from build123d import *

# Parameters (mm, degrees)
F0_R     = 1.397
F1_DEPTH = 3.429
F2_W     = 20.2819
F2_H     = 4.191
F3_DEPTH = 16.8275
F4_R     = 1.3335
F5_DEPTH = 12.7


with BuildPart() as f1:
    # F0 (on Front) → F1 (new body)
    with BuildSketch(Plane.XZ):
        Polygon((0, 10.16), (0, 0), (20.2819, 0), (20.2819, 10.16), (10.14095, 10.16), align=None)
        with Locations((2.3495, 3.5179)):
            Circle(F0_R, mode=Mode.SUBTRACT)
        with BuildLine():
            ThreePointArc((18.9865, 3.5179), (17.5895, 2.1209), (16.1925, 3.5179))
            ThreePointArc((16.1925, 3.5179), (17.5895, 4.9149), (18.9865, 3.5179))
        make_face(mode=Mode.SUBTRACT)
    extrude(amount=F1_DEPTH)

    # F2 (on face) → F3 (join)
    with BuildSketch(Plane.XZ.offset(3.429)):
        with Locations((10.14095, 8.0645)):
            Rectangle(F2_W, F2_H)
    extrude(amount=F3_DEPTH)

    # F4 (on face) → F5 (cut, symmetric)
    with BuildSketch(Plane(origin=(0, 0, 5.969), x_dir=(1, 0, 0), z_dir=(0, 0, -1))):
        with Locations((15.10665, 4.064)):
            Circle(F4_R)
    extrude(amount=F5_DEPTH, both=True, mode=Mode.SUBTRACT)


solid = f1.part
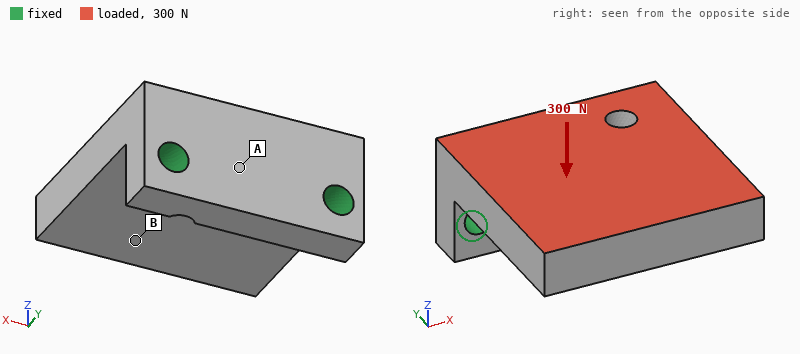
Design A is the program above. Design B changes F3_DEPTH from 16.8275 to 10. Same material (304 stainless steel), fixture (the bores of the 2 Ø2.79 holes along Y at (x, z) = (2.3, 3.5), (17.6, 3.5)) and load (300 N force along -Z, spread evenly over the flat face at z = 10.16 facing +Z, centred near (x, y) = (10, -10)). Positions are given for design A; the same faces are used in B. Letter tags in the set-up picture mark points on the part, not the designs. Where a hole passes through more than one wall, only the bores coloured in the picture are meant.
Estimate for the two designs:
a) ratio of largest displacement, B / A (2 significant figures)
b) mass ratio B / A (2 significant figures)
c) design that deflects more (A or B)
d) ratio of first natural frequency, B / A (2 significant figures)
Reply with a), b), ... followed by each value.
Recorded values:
a) 0.34
b) 0.72
c) A
d) 2.0
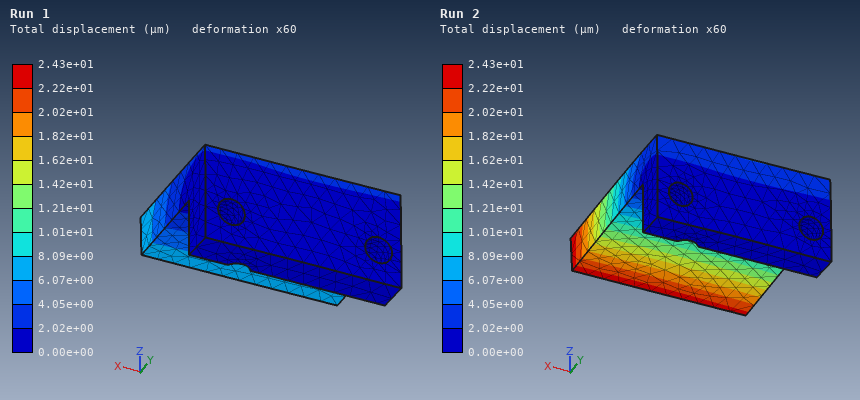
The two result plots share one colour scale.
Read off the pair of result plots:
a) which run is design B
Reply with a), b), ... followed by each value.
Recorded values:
a) Run 1
